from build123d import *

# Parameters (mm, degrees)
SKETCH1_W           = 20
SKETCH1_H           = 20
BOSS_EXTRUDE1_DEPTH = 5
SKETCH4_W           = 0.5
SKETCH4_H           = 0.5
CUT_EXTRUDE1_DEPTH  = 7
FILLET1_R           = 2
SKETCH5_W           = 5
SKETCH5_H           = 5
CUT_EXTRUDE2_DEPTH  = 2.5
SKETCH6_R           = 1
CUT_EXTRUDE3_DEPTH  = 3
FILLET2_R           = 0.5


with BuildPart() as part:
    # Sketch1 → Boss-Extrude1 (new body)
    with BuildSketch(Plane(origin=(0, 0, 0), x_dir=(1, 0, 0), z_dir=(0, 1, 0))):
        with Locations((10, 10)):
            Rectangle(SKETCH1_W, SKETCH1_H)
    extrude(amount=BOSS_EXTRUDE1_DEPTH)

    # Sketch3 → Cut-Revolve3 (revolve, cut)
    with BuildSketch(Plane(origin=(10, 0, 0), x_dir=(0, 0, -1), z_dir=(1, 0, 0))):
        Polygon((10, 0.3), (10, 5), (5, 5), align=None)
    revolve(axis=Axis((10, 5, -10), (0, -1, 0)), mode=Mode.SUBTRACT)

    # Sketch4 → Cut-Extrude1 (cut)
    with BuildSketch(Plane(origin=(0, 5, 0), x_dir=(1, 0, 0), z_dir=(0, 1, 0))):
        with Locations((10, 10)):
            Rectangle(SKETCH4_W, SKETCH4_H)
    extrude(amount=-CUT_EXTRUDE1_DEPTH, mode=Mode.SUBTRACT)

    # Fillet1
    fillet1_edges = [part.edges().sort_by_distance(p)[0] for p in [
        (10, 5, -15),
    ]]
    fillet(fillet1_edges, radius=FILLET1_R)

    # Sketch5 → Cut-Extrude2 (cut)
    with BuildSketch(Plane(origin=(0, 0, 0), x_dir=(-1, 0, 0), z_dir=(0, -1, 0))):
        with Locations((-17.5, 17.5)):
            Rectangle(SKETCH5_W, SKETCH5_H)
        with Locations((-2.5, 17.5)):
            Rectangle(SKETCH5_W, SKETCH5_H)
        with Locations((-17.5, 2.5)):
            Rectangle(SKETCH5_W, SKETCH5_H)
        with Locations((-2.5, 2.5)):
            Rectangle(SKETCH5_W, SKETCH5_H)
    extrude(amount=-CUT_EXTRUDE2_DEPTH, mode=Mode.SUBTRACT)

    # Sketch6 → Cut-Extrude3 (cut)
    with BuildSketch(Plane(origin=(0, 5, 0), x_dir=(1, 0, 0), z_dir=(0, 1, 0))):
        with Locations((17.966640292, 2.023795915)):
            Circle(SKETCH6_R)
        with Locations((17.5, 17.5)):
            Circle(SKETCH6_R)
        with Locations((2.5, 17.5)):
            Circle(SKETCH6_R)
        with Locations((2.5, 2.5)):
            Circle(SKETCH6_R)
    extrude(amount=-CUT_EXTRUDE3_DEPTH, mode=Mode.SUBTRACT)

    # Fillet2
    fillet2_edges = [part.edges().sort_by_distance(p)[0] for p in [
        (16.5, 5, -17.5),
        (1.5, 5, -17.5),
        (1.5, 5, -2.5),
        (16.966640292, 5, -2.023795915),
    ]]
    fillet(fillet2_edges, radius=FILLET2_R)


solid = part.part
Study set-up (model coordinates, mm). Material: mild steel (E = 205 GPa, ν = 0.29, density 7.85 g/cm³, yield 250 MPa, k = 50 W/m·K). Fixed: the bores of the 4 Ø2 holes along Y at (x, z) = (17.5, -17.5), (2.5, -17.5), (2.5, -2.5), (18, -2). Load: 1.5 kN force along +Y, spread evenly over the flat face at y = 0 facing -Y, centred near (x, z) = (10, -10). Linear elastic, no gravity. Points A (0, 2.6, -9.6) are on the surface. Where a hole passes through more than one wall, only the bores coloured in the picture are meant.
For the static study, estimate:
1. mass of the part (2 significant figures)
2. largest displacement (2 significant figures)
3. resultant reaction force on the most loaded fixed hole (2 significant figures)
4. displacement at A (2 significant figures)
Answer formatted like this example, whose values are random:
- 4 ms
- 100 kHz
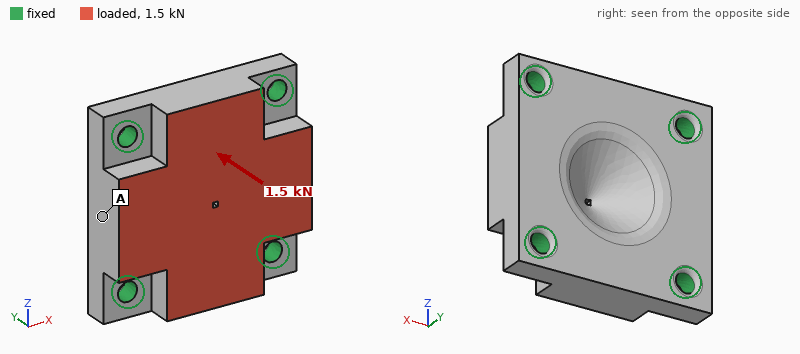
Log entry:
- 12 g
- 3.0 µm
- 440 N
- 1.5 µm
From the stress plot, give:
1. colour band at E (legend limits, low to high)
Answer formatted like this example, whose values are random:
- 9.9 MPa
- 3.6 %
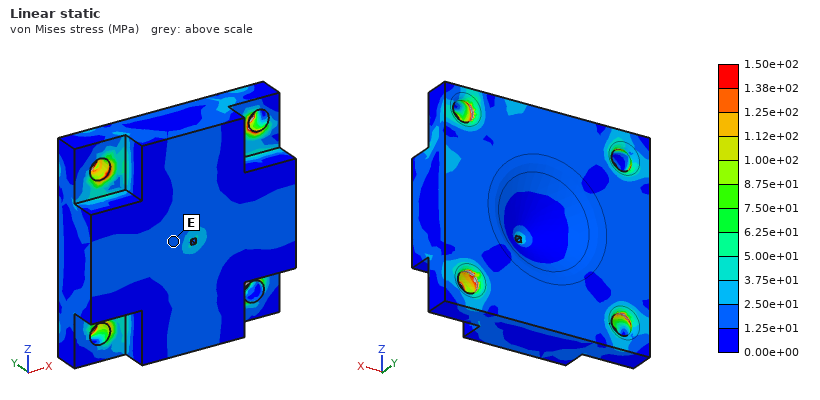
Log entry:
- 1.25e+01 to 2.50e+01 MPa
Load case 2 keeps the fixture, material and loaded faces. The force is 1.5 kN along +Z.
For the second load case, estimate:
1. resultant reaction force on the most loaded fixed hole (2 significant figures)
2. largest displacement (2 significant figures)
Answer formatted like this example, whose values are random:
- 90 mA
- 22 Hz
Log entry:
- 440 N
- 2.1 µm
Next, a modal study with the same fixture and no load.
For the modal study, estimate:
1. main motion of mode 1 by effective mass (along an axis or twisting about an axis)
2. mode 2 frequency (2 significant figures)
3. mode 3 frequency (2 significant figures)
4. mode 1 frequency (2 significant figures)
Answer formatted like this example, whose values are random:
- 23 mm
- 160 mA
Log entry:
- along Y
- 54 kHz
- 56 kHz
- 41 kHz
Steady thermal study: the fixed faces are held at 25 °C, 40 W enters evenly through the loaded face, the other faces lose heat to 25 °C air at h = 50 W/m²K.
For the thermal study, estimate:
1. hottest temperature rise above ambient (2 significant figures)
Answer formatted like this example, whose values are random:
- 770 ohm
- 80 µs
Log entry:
- 49 K
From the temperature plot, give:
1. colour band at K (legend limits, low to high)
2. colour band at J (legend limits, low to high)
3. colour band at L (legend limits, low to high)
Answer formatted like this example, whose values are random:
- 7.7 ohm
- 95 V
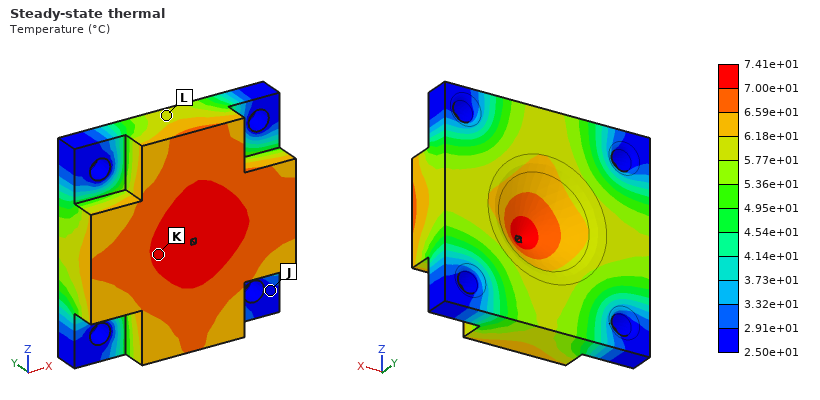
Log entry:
- 7.00e+01 to 7.41e+01 °C
- 2.50e+01 to 2.91e+01 °C
- 5.77e+01 to 6.18e+01 °C
